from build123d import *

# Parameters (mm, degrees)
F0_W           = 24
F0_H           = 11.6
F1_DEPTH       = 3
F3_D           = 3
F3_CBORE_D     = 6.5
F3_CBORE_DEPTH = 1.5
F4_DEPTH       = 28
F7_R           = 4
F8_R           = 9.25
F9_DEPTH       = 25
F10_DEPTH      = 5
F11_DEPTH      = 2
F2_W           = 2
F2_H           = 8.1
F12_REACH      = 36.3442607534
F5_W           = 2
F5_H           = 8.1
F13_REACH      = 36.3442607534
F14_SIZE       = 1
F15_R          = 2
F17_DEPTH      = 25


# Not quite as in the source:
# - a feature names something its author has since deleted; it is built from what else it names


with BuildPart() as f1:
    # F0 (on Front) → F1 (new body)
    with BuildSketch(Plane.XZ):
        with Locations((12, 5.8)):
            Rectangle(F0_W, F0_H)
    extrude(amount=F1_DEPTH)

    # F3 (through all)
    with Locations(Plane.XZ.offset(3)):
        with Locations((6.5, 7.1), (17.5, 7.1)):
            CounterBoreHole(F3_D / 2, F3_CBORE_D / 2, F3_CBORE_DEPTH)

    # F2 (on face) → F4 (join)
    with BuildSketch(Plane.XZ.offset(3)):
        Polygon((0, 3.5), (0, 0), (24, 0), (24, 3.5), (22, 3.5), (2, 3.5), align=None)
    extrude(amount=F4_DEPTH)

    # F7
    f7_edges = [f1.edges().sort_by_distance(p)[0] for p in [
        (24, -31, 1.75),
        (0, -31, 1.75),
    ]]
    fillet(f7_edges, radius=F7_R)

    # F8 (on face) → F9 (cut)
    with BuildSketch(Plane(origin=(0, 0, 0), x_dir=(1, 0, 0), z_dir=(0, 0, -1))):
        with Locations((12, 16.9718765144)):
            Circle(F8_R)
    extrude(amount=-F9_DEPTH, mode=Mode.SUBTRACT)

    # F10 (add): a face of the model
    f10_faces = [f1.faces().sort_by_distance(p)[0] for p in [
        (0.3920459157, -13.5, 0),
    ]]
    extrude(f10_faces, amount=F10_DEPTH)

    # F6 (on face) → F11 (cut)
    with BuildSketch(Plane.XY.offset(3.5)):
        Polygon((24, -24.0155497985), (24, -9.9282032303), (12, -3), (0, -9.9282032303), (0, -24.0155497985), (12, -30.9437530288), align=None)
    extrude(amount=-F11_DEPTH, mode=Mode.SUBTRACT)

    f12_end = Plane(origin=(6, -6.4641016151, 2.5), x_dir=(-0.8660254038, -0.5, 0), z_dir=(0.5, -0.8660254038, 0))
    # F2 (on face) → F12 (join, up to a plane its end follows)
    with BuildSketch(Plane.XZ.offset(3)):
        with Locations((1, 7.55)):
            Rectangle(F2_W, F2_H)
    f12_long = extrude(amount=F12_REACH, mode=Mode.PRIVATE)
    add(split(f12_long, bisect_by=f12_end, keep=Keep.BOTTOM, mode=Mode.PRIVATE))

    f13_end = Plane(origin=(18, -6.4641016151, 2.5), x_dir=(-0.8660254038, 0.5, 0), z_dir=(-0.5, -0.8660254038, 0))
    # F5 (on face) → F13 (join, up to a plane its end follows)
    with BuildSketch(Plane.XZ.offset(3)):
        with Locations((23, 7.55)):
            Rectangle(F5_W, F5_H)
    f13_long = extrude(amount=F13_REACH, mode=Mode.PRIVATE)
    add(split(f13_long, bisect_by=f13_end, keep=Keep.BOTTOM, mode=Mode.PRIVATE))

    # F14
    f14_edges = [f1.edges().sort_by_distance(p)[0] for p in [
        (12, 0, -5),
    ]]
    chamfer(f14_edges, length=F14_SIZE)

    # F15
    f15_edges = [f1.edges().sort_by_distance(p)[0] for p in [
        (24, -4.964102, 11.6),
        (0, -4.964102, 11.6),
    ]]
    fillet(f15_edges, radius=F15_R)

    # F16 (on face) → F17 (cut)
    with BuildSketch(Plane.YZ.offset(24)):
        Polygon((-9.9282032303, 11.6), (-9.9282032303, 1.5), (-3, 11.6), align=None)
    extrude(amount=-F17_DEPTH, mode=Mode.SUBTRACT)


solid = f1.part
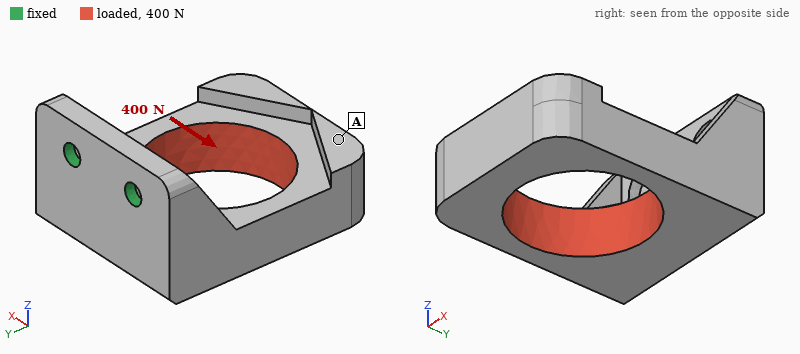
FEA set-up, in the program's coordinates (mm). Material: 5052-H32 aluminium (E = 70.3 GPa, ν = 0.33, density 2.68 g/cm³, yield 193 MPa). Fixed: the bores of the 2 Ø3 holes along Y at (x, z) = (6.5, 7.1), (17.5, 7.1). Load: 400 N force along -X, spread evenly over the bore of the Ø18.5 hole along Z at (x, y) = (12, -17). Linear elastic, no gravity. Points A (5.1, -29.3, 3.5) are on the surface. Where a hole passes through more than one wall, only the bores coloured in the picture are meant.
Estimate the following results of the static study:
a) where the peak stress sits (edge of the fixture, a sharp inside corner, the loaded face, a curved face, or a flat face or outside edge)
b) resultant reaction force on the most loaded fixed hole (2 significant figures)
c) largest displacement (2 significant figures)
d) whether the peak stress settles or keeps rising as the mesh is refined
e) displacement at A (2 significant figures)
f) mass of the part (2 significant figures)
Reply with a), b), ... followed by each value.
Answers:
a) edge of the fixture
b) 600 N
c) 0.10 mm
d) keeps rising
e) 0.097 mm
f) 11 g
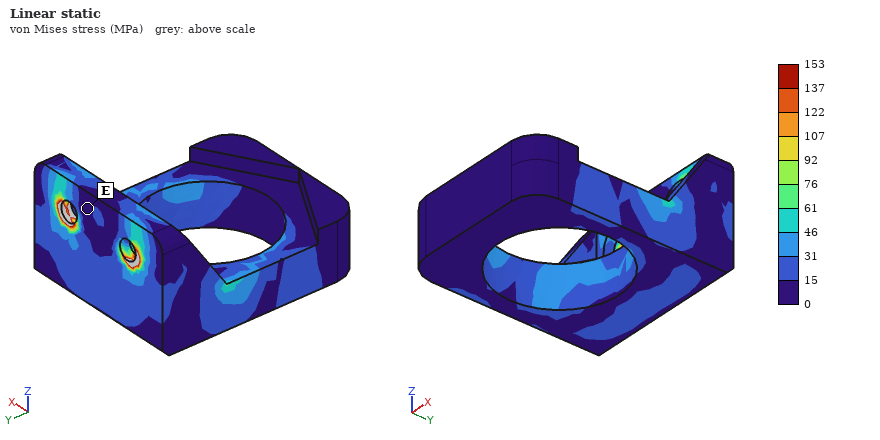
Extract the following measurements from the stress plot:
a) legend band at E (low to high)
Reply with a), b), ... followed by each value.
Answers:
a) 0 to 15 MPa
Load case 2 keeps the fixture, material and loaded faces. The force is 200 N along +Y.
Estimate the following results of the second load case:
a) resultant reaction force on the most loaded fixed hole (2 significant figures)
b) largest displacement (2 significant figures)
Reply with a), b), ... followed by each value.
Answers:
a) 100 N
b) 95 µm
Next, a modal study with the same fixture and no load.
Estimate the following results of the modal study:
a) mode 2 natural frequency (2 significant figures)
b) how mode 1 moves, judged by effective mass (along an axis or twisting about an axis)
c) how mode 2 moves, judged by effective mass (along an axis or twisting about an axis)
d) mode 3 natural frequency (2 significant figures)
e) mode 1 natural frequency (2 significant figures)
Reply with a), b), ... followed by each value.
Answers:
a) 4000 Hz
b) along Z
c) along X
d) 9300 Hz
e) 1900 Hz
